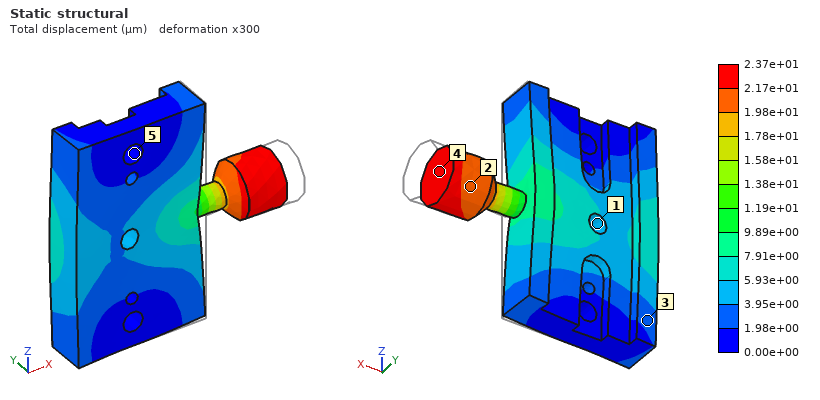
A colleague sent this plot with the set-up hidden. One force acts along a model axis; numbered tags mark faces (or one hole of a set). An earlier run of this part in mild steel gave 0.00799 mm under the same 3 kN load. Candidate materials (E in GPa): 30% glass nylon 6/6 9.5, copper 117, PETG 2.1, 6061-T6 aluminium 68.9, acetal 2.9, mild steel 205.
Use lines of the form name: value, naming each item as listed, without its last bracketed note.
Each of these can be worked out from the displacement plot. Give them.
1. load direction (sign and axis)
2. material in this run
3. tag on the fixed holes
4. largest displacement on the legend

load direction: -X
material in this run: 6061-T6 aluminium
tag on the fixed holes: 5
largest displacement on the legend: 2.37e+01 µm
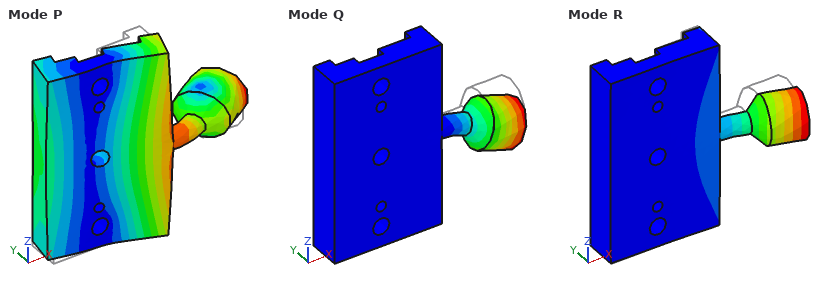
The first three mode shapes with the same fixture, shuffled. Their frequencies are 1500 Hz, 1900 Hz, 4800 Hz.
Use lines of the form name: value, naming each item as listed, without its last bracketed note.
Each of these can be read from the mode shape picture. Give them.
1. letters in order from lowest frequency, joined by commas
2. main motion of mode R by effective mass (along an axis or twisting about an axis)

letters in order from lowest frequency, joined by commas: R, Q, P
main motion of mode R by effective mass: along Y
